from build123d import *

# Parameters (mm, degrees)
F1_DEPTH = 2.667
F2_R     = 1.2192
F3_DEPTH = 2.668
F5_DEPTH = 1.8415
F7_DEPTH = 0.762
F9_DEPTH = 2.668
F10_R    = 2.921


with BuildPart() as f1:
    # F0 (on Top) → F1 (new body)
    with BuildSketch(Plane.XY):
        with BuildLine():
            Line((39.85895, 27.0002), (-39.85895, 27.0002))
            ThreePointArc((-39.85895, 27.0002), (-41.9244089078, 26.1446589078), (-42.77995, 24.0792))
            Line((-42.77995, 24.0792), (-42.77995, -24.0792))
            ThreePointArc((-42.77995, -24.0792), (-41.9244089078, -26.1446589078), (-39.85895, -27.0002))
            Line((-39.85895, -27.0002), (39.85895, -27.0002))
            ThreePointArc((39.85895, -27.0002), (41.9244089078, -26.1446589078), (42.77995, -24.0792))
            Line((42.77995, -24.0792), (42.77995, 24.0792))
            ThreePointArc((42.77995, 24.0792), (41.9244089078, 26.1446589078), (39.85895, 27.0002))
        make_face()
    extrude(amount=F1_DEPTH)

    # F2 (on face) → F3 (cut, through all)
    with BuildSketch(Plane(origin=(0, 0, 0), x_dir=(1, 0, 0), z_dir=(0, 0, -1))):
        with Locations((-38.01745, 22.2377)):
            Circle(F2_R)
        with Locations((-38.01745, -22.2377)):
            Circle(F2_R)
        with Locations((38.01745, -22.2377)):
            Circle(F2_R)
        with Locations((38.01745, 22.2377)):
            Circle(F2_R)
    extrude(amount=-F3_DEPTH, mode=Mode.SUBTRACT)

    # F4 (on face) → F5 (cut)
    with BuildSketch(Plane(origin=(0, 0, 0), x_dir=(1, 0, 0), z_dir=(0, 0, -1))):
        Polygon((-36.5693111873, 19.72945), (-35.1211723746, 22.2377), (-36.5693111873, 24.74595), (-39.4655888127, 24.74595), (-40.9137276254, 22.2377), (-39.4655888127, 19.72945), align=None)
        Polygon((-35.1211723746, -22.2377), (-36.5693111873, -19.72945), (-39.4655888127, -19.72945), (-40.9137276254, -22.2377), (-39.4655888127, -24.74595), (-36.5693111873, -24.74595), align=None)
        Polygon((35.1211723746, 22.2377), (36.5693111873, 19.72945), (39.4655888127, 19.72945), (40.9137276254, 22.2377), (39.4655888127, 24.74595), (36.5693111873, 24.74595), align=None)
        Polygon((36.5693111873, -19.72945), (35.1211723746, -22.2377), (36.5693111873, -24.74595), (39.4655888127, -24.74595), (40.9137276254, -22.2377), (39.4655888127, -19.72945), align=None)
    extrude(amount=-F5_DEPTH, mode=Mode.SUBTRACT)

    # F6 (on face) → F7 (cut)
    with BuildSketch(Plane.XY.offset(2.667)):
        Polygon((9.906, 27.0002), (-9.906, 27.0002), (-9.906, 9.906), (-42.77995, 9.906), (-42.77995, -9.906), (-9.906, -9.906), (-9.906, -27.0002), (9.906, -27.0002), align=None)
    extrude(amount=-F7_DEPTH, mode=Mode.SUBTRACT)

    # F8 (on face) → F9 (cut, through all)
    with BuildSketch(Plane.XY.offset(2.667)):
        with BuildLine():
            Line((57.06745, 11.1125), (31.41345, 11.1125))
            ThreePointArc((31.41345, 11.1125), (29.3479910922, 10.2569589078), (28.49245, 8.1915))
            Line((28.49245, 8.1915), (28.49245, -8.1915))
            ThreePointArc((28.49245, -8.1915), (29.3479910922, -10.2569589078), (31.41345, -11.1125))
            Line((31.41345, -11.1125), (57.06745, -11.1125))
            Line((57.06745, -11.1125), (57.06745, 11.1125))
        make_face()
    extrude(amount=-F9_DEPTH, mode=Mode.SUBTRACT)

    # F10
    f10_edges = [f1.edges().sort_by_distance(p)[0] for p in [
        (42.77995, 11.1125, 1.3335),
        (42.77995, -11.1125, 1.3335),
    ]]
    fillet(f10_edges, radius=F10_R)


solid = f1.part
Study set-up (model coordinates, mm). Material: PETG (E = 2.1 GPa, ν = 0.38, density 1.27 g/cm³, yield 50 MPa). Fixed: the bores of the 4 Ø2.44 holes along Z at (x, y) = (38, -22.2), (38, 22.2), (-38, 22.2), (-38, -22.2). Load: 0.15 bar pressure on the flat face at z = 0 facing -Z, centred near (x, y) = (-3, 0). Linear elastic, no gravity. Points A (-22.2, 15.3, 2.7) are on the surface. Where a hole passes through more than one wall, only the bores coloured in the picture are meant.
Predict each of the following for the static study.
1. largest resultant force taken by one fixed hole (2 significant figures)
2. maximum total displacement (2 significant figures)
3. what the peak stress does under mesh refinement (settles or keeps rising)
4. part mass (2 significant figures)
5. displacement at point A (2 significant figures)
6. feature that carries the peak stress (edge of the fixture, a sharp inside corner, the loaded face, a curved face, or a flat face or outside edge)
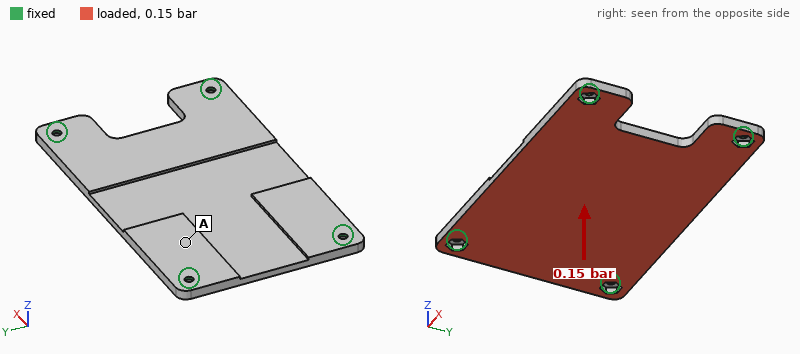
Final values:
81 N
1.2 mm
keeps rising
13 g
0.62 mm
edge of the fixture
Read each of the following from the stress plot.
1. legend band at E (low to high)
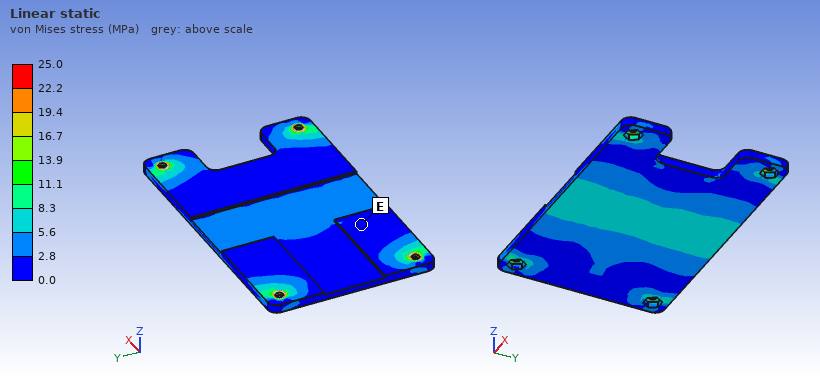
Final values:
0.0 to 2.8 MPa
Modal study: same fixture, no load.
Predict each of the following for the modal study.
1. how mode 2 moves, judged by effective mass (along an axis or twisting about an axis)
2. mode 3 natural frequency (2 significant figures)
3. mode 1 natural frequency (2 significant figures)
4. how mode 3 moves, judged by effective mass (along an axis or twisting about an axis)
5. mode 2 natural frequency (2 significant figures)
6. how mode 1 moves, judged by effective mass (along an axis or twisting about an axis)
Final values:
twisting about X
1000 Hz
390 Hz
twisting about Y
660 Hz
along Z
